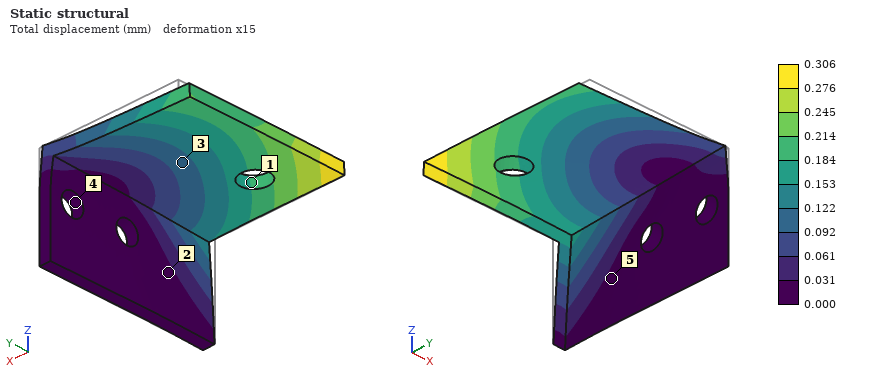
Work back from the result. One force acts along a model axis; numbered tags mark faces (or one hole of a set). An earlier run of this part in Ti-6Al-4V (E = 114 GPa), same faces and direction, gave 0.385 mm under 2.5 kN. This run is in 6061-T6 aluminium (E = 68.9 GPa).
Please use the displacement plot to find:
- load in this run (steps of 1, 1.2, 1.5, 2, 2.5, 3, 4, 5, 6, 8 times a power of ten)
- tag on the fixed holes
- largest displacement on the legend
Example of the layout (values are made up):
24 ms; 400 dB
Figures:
1.2 kN; 4; 0.306 mm
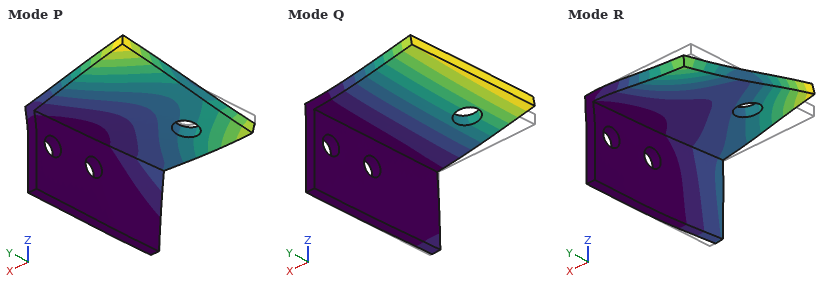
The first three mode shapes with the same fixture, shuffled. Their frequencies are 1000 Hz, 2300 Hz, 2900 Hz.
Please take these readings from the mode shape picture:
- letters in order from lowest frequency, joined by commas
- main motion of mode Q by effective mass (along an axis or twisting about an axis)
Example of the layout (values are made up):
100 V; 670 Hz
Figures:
Q, P, R; along Z
